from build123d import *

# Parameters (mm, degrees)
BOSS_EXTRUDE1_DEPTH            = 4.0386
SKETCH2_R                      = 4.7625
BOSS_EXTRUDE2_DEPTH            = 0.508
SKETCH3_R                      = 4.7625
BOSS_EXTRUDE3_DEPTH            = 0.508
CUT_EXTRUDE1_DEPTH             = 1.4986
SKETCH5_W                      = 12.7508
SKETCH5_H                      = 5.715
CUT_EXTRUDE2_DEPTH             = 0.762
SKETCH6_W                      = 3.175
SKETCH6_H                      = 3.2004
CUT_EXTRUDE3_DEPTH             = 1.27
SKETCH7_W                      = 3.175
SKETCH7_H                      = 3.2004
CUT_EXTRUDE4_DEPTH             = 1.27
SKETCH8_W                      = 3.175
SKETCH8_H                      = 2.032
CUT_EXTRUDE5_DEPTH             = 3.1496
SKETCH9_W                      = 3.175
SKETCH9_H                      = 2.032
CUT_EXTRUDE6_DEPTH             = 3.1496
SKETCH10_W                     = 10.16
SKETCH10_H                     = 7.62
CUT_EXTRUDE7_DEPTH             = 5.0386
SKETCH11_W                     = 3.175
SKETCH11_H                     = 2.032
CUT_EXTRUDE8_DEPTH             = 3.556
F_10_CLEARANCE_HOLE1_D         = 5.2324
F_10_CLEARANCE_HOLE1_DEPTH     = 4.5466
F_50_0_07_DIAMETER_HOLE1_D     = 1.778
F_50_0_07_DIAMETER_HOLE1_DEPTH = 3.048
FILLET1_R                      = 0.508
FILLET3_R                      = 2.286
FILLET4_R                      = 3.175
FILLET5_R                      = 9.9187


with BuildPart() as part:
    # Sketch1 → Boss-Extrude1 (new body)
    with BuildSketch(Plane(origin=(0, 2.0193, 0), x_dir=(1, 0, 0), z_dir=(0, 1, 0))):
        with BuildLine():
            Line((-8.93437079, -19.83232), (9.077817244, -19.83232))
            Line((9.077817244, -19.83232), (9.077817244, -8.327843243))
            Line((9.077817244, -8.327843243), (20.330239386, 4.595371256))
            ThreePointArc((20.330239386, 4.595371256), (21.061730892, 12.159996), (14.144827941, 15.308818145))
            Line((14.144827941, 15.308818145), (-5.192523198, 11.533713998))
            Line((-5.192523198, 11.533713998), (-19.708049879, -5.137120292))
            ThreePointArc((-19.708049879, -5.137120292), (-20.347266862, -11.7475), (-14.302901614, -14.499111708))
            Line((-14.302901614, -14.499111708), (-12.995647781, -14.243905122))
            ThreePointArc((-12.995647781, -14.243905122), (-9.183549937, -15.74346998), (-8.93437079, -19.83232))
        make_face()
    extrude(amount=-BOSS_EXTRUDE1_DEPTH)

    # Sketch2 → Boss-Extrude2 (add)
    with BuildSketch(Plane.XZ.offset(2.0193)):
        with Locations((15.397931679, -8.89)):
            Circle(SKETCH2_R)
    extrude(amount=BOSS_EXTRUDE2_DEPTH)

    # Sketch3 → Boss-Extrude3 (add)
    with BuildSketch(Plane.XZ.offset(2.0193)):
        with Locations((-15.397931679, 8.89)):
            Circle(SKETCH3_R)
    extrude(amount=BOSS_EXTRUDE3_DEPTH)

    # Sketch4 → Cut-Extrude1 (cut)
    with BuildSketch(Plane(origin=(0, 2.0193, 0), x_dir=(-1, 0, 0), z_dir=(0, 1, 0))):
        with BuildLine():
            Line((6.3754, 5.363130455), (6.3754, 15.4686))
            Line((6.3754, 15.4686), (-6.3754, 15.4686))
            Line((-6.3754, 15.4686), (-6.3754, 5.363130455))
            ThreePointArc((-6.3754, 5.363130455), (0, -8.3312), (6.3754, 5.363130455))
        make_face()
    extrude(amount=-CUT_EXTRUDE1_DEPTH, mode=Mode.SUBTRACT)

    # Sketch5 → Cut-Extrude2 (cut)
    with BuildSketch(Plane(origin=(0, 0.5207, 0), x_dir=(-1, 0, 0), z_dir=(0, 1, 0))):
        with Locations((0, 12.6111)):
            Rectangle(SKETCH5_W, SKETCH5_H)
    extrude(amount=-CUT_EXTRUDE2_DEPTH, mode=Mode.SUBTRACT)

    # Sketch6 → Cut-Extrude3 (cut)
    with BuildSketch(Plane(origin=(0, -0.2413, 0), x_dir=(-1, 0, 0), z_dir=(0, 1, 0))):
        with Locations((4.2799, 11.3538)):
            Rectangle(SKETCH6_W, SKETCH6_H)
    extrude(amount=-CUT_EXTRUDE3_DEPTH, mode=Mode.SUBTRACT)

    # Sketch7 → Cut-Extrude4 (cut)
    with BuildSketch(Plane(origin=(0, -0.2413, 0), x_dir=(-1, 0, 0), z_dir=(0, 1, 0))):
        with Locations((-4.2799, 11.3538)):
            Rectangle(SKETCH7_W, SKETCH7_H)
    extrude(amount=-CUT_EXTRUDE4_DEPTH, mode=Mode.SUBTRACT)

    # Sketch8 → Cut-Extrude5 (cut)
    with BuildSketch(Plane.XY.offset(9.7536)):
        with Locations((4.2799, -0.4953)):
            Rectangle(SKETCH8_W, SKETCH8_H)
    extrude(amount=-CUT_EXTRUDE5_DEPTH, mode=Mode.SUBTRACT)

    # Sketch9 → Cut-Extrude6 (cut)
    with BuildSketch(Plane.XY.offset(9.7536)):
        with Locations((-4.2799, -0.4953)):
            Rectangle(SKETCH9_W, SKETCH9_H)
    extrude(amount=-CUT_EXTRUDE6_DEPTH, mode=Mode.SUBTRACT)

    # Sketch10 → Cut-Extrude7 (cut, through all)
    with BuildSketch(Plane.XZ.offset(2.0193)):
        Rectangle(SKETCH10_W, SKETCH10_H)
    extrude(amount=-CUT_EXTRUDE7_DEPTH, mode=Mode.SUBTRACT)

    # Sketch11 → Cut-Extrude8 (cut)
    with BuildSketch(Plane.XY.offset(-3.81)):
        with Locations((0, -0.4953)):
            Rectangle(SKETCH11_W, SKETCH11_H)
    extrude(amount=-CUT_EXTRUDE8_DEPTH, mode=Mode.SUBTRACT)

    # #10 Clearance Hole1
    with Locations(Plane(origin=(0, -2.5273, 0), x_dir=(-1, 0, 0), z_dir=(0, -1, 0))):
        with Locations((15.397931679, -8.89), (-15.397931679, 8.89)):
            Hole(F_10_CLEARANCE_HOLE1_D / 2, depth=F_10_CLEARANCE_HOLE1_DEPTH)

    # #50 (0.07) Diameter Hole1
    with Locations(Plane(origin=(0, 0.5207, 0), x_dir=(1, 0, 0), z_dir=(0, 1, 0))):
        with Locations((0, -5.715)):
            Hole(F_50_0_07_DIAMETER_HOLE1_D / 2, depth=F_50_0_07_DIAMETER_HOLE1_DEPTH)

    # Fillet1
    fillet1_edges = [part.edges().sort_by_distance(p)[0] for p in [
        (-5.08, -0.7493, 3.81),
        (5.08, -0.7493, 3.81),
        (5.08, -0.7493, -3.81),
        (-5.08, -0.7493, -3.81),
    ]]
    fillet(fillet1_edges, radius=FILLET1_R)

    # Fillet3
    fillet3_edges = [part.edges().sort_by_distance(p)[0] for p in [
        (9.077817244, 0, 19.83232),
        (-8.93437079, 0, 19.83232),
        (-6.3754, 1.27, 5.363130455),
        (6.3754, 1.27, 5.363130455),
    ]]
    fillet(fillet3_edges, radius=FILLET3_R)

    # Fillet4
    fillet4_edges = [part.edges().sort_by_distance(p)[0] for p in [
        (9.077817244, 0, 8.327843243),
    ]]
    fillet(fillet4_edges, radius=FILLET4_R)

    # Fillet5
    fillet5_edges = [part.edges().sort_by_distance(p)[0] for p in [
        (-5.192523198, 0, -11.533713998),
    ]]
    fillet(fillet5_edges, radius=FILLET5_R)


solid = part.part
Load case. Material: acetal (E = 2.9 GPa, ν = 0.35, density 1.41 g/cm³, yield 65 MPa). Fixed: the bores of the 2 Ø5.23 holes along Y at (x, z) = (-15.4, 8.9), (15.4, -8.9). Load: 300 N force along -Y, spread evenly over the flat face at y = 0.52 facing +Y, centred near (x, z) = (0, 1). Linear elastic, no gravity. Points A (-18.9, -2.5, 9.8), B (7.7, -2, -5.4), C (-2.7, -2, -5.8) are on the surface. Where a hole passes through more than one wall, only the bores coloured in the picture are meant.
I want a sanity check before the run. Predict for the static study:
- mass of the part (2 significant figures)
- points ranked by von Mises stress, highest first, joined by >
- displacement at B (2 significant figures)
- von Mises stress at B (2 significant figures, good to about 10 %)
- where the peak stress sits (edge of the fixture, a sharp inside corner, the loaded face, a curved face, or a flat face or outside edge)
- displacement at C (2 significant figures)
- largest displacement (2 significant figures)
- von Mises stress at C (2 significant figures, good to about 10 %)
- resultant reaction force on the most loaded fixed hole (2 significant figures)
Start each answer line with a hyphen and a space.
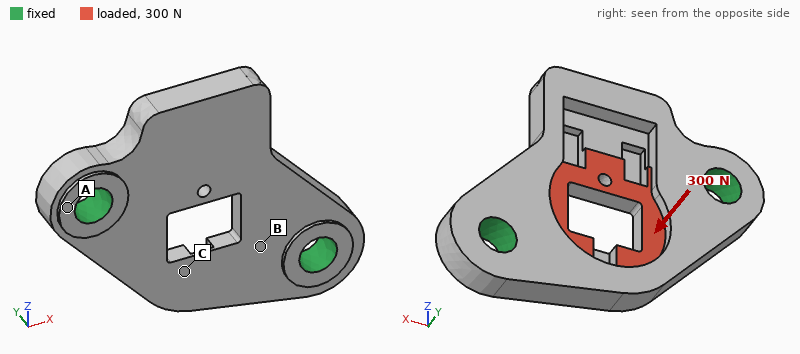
- 4.0 g
- C > B > A
- 0.11 mm
- 10 MPa
- a curved face
- 0.23 mm
- 0.38 mm
- 18 MPa
- 160 N
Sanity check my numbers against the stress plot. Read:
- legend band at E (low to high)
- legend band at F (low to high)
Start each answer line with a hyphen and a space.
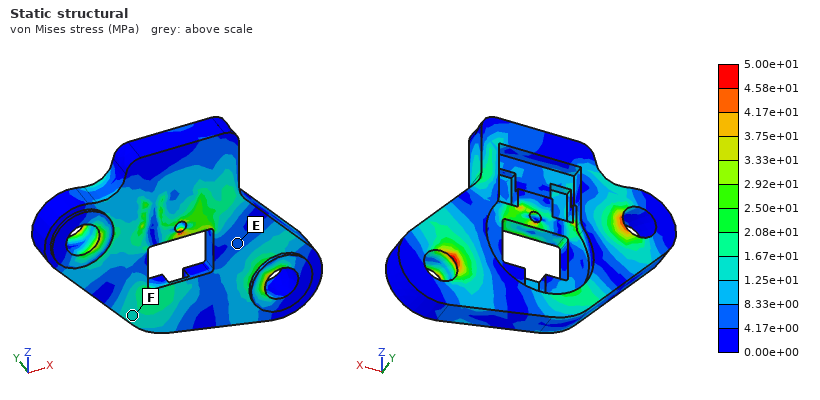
- 4.17e+00 to 8.33e+00 MPa
- 1.25e+01 to 1.67e+01 MPa
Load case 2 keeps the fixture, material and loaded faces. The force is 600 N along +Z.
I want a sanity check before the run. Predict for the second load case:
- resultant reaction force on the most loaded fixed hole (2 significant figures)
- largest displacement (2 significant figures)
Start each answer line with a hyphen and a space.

- 300 N
- 0.16 mm
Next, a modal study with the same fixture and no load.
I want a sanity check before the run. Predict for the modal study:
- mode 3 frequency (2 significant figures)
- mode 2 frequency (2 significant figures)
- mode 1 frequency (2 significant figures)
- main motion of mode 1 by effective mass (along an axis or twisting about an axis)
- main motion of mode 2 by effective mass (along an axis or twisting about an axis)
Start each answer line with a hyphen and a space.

- 6200 Hz
- 4600 Hz
- 2400 Hz
- along Y
- along Y
